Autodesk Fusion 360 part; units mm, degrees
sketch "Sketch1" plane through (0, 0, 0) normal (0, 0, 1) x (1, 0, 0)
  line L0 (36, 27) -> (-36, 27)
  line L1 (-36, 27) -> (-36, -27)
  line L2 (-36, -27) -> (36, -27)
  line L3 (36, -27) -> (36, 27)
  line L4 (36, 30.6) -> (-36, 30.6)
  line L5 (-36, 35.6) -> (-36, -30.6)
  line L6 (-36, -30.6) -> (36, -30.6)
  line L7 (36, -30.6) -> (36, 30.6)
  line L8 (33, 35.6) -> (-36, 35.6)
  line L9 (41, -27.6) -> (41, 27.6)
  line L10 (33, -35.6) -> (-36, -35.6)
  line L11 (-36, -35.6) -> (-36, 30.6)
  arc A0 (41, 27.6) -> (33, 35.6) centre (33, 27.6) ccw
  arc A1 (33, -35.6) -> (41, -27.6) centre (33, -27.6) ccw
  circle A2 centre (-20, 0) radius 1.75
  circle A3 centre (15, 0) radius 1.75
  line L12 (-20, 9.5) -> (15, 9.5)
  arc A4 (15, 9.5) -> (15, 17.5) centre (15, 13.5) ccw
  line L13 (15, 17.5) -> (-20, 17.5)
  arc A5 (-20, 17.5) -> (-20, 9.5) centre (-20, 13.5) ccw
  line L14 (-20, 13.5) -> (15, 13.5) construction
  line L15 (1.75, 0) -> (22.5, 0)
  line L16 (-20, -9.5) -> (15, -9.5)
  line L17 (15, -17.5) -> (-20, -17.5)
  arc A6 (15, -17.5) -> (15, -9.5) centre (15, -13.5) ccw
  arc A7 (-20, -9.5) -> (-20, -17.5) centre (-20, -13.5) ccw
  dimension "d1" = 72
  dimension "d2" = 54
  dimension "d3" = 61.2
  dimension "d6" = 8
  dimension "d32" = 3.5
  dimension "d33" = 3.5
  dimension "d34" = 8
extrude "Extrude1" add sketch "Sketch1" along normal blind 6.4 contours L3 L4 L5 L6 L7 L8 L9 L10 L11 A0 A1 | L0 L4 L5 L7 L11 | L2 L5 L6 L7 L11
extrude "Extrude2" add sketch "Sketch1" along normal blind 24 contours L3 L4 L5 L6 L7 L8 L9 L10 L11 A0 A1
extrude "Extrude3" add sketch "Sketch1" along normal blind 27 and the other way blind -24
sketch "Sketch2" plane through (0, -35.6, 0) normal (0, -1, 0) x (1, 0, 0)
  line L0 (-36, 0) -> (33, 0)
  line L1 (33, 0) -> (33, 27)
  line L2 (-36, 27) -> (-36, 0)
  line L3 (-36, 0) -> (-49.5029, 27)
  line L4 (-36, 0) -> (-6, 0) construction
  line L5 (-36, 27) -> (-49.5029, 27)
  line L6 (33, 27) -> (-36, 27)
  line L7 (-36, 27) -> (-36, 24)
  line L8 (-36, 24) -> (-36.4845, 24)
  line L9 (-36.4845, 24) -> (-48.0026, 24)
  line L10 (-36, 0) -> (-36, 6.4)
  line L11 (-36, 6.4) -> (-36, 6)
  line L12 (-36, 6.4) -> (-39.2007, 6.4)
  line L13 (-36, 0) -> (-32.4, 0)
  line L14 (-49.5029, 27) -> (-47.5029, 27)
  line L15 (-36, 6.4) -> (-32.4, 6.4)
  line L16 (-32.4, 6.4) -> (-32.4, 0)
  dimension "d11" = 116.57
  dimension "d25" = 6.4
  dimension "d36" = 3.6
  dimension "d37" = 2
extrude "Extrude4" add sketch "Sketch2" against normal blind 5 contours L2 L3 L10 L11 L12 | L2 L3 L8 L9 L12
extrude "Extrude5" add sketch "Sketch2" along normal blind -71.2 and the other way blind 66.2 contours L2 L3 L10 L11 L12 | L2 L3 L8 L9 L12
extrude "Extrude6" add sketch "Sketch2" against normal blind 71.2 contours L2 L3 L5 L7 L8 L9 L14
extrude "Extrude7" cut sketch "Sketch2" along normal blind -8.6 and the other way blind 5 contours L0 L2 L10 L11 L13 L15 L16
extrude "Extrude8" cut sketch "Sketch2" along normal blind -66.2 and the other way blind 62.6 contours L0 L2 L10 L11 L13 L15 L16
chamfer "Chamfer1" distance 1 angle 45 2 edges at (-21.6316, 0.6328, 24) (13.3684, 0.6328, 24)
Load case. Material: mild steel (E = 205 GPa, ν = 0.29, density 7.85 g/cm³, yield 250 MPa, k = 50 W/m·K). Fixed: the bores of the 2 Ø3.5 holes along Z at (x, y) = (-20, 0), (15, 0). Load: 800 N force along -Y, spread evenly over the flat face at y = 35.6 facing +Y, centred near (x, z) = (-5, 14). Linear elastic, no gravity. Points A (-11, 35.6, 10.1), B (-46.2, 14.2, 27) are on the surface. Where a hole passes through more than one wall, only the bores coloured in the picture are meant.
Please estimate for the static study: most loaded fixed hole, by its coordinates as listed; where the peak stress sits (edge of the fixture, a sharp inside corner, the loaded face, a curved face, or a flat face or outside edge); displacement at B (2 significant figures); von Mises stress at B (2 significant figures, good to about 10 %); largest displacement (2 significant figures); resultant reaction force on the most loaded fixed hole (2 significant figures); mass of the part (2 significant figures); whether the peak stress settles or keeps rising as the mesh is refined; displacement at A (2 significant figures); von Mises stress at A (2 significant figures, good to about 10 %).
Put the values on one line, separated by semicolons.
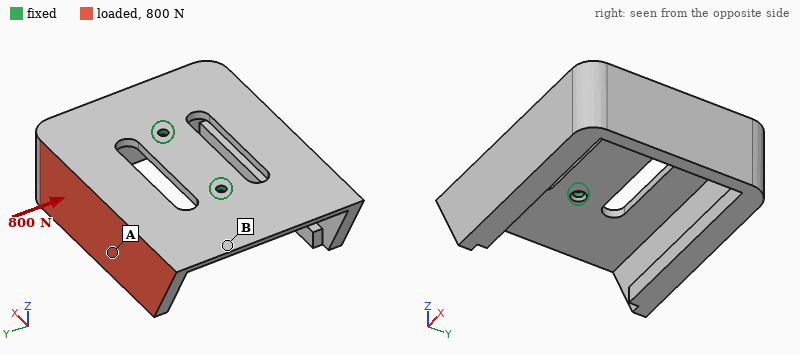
(-20, 0); edge of the fixture; 0.049 mm; 44 MPa; 0.25 mm; 470 N; 370 g; keeps rising; 0.21 mm; 16 MPa
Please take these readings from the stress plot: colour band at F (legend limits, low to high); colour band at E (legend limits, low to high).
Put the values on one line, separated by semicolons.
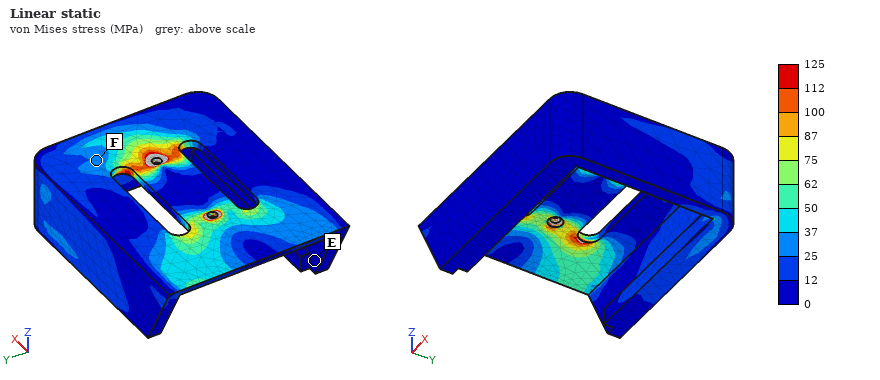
25 to 37 MPa; 0 to 12 MPa
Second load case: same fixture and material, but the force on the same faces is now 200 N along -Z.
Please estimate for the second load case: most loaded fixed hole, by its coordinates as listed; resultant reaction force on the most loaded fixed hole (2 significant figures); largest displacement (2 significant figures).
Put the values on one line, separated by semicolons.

(-20, 0); 120 N; 0.17 mm
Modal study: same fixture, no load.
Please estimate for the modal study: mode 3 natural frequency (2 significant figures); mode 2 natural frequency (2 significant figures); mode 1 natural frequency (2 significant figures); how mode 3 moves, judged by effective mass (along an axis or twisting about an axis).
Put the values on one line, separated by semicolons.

1200 Hz; 950 Hz; 410 Hz; along Z
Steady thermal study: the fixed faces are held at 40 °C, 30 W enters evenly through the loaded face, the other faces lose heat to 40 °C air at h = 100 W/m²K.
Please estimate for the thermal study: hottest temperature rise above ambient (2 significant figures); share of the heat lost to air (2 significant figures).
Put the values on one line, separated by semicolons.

43 K; 89 %
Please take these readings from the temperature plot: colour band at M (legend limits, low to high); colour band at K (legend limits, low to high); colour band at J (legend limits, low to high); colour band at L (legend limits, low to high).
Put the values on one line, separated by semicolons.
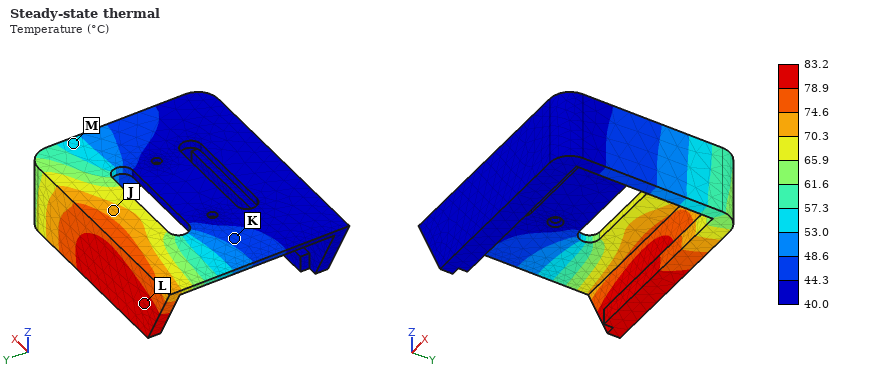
53.0 to 57.3 °C; 44.3 to 48.6 °C; 70.3 to 74.6 °C; 78.9 to 83.2 °C
